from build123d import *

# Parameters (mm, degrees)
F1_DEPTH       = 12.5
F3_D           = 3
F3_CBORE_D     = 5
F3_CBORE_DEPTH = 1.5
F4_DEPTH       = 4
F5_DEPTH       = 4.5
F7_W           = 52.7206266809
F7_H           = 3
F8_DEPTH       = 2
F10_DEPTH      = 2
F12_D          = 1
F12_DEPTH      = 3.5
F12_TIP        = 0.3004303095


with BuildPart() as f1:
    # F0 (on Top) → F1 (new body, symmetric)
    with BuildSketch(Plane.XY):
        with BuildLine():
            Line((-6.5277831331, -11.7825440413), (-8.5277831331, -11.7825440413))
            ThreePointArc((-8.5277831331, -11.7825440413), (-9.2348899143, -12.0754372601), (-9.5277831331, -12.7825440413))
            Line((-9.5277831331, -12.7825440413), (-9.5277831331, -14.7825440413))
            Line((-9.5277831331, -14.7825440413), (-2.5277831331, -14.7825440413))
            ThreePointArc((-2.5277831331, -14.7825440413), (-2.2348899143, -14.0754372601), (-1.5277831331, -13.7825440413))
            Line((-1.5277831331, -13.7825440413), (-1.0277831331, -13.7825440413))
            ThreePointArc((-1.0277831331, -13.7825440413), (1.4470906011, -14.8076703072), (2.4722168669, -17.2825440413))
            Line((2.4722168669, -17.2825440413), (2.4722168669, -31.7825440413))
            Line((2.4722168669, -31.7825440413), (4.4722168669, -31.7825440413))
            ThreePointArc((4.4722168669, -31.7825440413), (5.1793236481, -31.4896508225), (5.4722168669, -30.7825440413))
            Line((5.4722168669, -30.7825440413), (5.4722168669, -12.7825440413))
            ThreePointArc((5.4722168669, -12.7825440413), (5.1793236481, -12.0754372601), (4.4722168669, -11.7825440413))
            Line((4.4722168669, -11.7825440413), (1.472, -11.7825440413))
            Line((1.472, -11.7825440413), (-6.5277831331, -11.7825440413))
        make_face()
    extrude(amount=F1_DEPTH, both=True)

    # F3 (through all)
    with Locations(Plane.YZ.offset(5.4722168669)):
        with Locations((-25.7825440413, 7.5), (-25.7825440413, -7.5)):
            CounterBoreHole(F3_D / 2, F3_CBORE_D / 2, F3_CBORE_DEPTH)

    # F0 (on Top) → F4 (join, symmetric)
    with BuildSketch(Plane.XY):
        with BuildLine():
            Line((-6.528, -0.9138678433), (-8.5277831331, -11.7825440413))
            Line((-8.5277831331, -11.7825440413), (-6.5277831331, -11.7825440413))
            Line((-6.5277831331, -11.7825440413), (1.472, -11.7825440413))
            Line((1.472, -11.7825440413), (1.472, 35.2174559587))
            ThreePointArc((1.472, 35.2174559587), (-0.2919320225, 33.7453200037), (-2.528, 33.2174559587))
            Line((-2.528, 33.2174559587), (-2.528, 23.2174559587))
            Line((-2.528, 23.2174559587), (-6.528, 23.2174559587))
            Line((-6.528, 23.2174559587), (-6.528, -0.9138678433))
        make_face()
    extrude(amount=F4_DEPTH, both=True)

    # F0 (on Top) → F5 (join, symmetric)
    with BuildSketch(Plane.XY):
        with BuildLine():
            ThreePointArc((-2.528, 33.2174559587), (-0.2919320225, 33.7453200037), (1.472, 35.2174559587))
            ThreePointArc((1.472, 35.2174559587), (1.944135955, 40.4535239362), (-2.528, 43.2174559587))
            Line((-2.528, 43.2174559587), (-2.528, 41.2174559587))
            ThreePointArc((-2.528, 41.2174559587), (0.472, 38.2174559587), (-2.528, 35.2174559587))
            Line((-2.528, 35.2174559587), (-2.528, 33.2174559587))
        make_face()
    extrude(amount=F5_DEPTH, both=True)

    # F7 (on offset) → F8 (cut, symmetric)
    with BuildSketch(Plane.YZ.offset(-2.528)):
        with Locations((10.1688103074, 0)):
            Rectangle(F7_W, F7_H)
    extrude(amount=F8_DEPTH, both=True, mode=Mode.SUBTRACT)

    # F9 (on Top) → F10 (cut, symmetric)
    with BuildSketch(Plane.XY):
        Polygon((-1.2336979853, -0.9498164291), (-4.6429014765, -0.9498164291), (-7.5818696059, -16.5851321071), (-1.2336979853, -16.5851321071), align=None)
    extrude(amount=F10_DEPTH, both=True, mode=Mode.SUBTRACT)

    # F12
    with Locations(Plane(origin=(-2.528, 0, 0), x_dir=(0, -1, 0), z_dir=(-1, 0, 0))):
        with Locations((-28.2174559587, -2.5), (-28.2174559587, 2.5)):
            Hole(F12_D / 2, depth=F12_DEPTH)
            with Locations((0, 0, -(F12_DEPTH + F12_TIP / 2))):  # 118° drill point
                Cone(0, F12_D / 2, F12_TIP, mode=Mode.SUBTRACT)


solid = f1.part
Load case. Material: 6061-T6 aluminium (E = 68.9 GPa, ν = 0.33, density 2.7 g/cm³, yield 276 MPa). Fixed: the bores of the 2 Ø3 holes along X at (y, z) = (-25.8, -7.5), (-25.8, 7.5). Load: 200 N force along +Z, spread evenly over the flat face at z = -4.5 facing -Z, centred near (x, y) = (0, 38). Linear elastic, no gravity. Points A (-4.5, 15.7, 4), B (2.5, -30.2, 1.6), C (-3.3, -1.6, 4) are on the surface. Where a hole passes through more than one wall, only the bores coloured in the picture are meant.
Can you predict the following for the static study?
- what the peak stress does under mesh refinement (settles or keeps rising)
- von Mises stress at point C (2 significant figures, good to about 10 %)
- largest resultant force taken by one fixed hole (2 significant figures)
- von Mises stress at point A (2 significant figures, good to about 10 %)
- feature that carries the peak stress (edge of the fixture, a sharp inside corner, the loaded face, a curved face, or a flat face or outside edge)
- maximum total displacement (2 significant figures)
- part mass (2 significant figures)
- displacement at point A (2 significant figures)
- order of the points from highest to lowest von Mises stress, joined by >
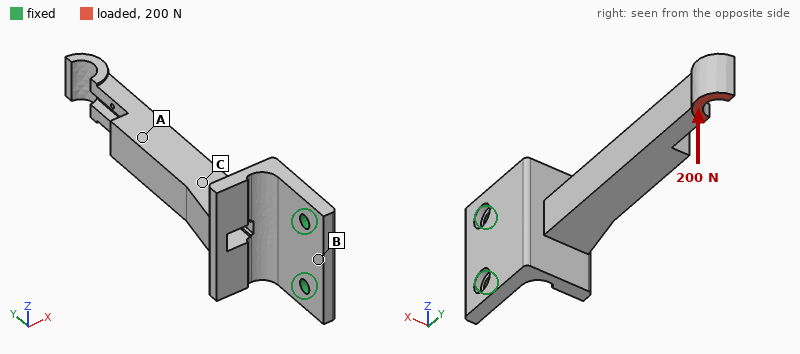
keeps rising
93 MPa
790 N
48 MPa
a sharp inside corner
0.86 mm
12 g
0.33 mm
C > A > B
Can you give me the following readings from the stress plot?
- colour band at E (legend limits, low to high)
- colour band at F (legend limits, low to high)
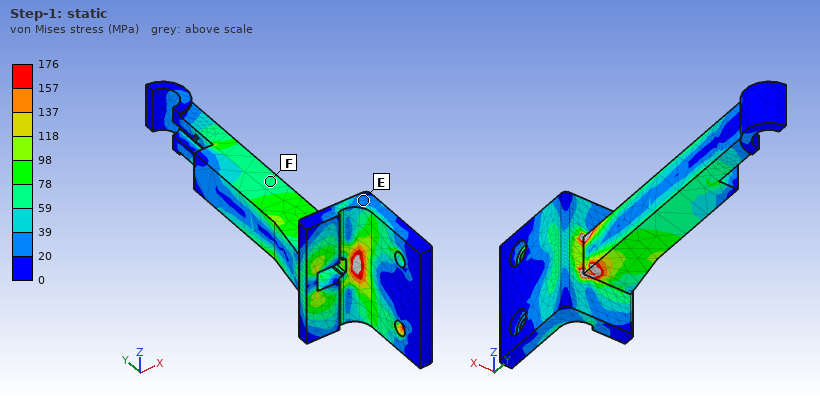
20 to 39 MPa
59 to 78 MPa
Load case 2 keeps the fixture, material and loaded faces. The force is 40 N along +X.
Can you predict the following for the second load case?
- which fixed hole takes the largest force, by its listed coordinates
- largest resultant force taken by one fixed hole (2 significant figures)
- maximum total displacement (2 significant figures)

(-25.8, -7.5)
43 N
0.94 mm
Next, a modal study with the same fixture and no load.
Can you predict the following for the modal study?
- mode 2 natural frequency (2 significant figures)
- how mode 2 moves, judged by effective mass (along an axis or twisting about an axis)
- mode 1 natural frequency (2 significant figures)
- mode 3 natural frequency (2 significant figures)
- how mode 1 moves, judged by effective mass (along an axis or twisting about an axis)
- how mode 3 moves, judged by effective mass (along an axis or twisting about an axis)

2100 Hz
along Z
750 Hz
5300 Hz
along X
along X
